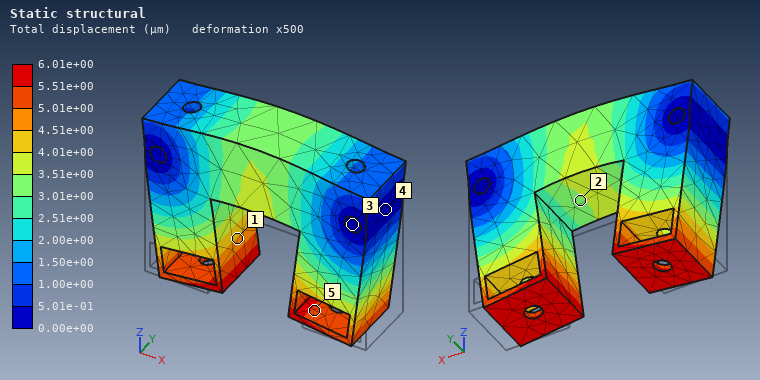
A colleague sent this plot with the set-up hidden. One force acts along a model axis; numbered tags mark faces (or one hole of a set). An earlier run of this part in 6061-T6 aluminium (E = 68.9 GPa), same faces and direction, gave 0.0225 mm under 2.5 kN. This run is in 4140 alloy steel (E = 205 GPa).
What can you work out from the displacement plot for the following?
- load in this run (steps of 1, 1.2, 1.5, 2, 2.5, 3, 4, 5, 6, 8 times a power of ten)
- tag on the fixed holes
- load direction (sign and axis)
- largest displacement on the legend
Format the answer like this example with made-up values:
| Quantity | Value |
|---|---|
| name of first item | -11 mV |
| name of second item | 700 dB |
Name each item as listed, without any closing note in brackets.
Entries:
| Quantity | Value |
|---|---|
| load in this run | 2 kN |
| tag on the fixed holes | 3 |
| load direction | +Z |
| largest displacement on the legend | 6.01e+00 µm |
